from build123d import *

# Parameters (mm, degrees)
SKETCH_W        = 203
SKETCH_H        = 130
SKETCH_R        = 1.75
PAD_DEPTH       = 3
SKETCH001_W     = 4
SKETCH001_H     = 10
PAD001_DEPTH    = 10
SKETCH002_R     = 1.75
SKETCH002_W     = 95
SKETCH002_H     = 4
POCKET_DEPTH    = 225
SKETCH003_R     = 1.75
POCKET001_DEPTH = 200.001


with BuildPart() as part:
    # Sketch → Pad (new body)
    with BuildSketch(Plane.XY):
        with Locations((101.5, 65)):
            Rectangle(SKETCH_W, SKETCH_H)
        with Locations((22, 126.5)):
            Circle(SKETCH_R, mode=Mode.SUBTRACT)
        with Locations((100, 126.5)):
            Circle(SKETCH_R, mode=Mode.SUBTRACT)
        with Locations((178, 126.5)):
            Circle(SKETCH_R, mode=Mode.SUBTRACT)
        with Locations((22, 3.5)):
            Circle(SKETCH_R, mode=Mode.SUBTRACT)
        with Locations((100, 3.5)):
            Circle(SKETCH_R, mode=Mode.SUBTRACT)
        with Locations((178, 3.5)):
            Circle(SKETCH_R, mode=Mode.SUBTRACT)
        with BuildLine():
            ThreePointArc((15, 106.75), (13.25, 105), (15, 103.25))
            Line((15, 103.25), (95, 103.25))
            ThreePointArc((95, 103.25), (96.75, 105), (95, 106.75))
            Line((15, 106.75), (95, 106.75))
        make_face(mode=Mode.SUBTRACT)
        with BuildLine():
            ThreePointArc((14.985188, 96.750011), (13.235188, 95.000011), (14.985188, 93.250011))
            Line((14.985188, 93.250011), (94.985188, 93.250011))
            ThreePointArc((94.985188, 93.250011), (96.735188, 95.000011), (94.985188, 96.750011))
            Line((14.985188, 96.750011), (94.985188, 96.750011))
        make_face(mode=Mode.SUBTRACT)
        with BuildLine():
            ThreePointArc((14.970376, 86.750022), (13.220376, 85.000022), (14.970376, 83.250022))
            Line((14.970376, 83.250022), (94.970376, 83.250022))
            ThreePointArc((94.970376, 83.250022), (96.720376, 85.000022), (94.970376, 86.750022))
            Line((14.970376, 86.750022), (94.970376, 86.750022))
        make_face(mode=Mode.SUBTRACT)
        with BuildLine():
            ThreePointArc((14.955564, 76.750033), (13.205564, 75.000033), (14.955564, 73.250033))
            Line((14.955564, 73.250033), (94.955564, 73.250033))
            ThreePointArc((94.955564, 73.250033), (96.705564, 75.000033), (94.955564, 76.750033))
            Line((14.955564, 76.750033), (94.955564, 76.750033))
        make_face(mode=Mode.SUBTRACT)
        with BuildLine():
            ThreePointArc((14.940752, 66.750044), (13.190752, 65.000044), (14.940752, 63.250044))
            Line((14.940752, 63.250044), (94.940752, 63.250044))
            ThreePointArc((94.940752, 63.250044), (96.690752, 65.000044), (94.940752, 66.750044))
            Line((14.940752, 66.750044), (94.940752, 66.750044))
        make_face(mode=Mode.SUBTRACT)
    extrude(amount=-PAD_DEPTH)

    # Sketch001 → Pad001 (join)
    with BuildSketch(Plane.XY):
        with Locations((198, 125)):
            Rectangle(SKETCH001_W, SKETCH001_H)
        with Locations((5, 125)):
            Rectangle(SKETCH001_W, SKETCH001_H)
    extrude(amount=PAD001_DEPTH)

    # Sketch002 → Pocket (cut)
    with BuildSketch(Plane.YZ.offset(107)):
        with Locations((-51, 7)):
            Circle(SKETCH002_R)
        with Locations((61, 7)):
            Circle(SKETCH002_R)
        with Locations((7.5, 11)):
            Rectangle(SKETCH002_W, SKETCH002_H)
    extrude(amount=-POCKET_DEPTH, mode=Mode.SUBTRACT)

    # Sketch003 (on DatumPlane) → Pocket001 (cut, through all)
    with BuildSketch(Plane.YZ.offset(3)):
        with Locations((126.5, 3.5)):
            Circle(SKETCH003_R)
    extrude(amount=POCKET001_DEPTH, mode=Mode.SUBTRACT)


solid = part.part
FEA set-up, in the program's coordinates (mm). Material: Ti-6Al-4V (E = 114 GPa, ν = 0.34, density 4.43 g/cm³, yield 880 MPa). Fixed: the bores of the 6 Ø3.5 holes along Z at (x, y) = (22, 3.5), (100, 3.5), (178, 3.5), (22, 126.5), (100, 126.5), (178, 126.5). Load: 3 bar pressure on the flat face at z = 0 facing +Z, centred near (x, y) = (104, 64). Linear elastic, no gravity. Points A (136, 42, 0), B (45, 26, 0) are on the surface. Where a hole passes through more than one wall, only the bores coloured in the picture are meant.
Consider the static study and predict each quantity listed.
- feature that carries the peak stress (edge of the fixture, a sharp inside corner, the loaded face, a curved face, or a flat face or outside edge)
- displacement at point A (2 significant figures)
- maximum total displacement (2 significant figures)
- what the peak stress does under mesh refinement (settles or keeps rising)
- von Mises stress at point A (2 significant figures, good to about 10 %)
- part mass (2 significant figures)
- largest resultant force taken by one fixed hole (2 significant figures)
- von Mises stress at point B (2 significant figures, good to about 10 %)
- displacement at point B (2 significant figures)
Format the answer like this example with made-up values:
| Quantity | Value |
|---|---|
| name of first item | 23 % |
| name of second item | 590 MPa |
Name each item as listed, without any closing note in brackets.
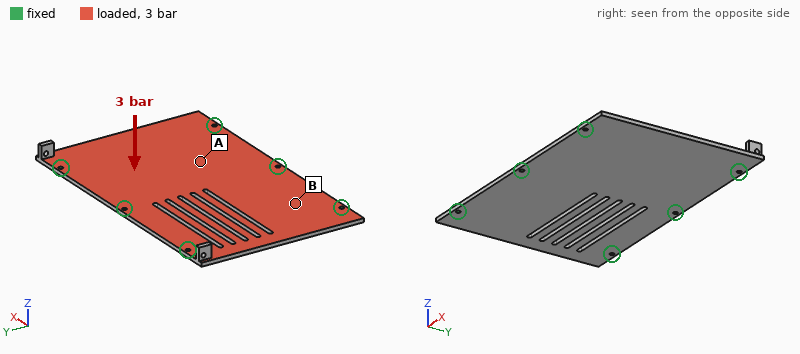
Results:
| Quantity | Value |
|---|---|
| feature that carries the peak stress | edge of the fixture |
| displacement at point A | 1.0 mm |
| maximum total displacement | 2.2 mm |
| what the peak stress does under mesh refinement | keeps rising |
| von Mises stress at point A | 110 MPa |
| part mass | 330 g |
| largest resultant force taken by one fixed hole | 1.5 kN |
| von Mises stress at point B | 56 MPa |
| displacement at point B | 0.74 mm |
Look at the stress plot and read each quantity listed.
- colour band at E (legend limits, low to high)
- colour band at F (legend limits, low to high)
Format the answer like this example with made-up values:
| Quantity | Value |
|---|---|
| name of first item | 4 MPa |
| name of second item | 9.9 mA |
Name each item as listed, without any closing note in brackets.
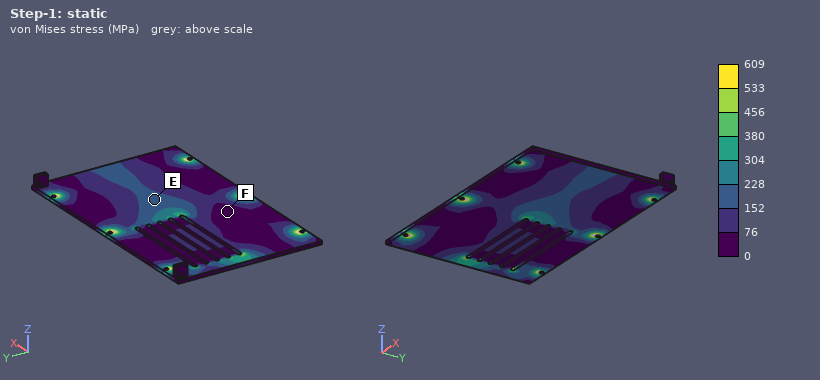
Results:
| Quantity | Value |
|---|---|
| colour band at E | 152 to 228 MPa |
| colour band at F | 0 to 76 MPa |
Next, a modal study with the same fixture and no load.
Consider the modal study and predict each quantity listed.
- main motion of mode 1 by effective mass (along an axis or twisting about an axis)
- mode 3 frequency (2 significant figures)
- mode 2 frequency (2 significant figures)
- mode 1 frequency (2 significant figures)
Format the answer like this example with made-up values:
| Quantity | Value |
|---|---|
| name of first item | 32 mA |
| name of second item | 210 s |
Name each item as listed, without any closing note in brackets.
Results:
| Quantity | Value |
|---|---|
| main motion of mode 1 by effective mass | along Z |
| mode 3 frequency | 1100 Hz |
| mode 2 frequency | 870 Hz |
| mode 1 frequency | 660 Hz |
